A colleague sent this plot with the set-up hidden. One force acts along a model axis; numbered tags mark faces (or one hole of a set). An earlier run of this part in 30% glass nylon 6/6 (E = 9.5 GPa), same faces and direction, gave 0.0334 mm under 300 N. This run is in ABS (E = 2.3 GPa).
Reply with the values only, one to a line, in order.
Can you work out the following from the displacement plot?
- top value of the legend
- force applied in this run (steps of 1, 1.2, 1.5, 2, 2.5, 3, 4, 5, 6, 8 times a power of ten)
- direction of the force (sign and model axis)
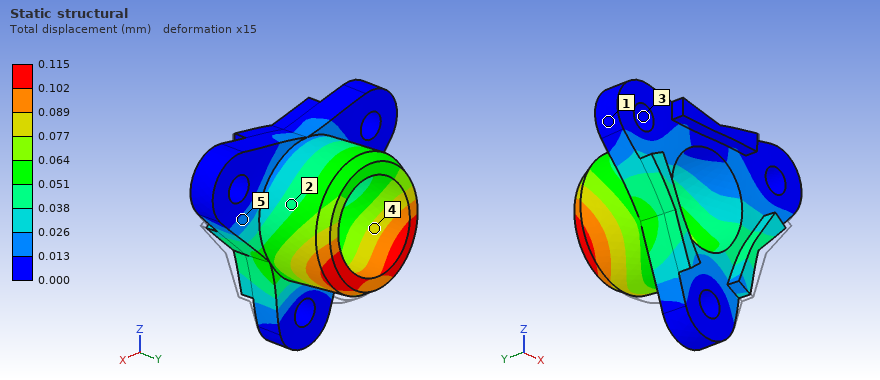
0.115 mm
250 N
-X
